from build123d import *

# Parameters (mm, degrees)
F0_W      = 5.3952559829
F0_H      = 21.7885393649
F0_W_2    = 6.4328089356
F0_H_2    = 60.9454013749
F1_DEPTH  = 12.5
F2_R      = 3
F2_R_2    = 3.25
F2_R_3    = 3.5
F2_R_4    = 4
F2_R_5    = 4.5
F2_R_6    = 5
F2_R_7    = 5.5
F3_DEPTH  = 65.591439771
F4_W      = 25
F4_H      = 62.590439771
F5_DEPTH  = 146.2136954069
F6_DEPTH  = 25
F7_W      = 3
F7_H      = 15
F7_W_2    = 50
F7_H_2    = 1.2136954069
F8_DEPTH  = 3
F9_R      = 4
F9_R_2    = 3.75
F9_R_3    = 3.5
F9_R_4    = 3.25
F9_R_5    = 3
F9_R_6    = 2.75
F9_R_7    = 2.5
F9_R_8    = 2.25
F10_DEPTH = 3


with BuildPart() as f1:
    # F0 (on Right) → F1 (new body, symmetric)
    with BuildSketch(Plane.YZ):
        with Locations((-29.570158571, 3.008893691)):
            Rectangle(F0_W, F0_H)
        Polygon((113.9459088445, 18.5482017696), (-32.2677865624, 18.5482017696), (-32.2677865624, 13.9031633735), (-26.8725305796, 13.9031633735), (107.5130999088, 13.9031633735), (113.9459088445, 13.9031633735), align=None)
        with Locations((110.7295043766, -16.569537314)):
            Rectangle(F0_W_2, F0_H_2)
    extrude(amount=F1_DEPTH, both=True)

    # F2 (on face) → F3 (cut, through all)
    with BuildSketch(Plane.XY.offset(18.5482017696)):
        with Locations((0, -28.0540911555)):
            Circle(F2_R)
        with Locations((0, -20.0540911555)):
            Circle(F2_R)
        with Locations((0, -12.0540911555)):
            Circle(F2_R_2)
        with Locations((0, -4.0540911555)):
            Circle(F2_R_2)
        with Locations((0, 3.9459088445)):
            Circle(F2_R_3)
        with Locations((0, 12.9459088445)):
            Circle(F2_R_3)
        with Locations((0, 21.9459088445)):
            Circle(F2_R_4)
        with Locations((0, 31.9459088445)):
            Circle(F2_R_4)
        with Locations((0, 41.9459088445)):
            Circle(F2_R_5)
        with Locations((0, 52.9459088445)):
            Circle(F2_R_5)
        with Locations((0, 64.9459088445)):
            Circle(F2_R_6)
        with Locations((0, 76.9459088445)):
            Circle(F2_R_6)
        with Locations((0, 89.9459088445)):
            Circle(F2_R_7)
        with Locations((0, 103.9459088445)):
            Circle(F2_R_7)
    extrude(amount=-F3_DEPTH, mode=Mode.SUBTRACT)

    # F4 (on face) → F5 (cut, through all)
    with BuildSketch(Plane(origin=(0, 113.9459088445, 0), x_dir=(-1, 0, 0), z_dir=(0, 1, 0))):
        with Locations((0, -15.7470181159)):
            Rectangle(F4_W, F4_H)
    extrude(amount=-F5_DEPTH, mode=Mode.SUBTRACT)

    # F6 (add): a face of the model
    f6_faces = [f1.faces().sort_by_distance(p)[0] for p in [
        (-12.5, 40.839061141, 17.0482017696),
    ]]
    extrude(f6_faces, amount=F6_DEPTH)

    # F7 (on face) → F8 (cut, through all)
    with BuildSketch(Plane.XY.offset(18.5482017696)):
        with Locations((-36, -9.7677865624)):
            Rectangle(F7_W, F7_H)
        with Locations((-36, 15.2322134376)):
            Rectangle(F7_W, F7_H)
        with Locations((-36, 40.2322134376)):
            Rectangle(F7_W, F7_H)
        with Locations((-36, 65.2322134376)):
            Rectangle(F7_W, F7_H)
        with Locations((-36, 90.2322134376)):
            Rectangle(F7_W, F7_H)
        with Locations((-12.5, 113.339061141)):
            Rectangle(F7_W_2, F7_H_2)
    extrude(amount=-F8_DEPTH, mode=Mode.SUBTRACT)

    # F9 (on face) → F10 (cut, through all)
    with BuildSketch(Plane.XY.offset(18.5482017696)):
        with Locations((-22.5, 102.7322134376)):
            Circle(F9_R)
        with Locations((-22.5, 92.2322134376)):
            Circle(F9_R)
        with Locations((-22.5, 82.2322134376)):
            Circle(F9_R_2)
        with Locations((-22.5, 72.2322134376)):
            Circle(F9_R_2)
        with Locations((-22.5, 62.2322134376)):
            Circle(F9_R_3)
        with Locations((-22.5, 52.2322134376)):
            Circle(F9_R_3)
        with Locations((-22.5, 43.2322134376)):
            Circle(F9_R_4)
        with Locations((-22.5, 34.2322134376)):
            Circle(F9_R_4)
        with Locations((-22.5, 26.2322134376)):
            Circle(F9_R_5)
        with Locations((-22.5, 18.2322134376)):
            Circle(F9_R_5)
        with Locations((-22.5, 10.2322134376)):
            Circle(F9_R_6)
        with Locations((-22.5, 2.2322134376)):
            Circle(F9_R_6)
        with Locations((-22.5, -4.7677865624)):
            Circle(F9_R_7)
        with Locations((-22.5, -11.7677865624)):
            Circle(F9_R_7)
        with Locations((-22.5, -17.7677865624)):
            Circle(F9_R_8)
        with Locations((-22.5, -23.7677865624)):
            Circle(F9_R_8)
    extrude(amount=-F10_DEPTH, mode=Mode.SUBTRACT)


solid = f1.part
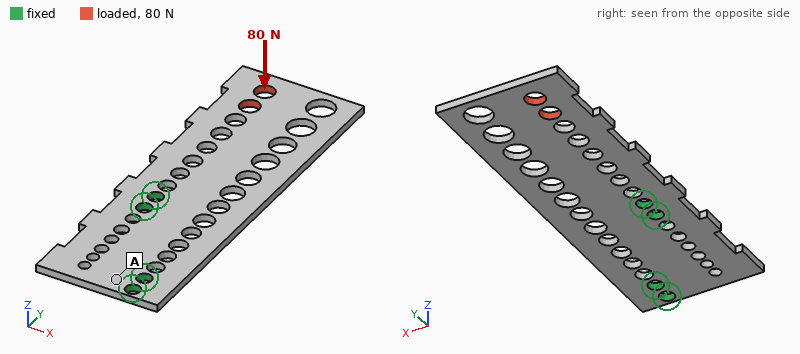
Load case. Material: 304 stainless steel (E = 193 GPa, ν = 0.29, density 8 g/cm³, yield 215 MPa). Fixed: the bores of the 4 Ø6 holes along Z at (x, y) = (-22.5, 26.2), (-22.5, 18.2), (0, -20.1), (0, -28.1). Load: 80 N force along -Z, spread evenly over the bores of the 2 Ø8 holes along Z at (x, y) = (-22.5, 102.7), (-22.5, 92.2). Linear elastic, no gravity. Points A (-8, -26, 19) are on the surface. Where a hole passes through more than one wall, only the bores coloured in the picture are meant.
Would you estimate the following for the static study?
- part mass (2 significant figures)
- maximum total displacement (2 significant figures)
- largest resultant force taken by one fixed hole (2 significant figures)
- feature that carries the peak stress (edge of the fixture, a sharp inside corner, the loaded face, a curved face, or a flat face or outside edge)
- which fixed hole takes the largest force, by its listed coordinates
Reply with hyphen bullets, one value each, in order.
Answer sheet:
- 140 g
- 0.93 mm
- 310 N
- a curved face
- (-22.5, 26.2)
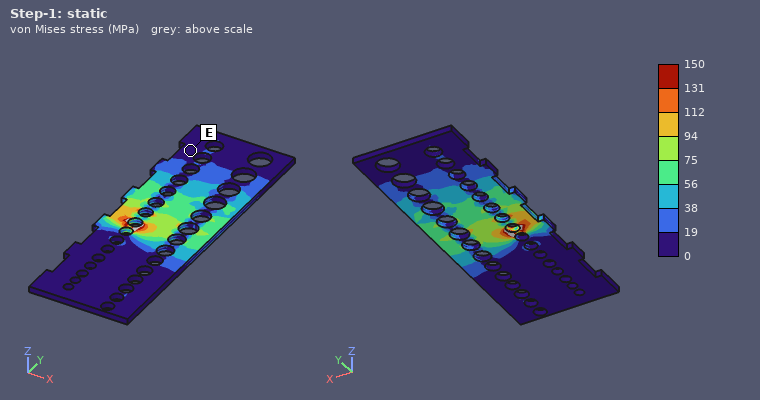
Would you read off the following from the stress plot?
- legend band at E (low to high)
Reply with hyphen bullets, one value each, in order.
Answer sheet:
- 0 to 19 MPa
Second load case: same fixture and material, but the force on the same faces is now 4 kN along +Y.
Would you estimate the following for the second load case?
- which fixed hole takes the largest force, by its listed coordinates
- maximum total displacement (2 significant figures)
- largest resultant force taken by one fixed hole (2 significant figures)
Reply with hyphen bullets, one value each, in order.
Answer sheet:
- (-22.5, 26.2)
- 52 µm
- 2.5 kN
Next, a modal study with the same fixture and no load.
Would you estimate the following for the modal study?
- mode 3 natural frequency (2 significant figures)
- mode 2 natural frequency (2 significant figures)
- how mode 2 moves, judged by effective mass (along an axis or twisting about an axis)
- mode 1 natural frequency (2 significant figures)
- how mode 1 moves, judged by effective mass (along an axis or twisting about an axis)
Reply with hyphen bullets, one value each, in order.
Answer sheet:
- 1700 Hz
- 940 Hz
- twisting about Y
- 290 Hz
- along Z
